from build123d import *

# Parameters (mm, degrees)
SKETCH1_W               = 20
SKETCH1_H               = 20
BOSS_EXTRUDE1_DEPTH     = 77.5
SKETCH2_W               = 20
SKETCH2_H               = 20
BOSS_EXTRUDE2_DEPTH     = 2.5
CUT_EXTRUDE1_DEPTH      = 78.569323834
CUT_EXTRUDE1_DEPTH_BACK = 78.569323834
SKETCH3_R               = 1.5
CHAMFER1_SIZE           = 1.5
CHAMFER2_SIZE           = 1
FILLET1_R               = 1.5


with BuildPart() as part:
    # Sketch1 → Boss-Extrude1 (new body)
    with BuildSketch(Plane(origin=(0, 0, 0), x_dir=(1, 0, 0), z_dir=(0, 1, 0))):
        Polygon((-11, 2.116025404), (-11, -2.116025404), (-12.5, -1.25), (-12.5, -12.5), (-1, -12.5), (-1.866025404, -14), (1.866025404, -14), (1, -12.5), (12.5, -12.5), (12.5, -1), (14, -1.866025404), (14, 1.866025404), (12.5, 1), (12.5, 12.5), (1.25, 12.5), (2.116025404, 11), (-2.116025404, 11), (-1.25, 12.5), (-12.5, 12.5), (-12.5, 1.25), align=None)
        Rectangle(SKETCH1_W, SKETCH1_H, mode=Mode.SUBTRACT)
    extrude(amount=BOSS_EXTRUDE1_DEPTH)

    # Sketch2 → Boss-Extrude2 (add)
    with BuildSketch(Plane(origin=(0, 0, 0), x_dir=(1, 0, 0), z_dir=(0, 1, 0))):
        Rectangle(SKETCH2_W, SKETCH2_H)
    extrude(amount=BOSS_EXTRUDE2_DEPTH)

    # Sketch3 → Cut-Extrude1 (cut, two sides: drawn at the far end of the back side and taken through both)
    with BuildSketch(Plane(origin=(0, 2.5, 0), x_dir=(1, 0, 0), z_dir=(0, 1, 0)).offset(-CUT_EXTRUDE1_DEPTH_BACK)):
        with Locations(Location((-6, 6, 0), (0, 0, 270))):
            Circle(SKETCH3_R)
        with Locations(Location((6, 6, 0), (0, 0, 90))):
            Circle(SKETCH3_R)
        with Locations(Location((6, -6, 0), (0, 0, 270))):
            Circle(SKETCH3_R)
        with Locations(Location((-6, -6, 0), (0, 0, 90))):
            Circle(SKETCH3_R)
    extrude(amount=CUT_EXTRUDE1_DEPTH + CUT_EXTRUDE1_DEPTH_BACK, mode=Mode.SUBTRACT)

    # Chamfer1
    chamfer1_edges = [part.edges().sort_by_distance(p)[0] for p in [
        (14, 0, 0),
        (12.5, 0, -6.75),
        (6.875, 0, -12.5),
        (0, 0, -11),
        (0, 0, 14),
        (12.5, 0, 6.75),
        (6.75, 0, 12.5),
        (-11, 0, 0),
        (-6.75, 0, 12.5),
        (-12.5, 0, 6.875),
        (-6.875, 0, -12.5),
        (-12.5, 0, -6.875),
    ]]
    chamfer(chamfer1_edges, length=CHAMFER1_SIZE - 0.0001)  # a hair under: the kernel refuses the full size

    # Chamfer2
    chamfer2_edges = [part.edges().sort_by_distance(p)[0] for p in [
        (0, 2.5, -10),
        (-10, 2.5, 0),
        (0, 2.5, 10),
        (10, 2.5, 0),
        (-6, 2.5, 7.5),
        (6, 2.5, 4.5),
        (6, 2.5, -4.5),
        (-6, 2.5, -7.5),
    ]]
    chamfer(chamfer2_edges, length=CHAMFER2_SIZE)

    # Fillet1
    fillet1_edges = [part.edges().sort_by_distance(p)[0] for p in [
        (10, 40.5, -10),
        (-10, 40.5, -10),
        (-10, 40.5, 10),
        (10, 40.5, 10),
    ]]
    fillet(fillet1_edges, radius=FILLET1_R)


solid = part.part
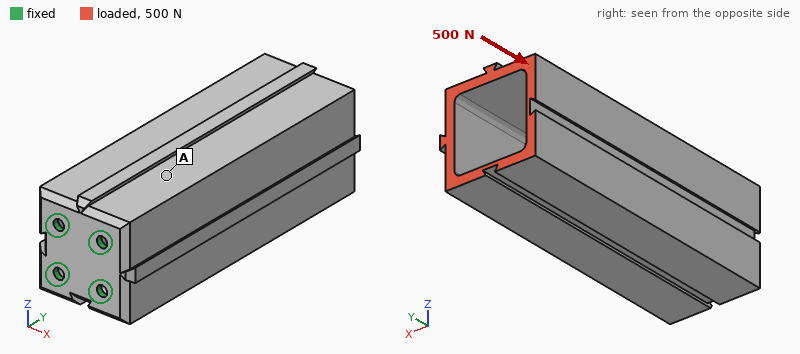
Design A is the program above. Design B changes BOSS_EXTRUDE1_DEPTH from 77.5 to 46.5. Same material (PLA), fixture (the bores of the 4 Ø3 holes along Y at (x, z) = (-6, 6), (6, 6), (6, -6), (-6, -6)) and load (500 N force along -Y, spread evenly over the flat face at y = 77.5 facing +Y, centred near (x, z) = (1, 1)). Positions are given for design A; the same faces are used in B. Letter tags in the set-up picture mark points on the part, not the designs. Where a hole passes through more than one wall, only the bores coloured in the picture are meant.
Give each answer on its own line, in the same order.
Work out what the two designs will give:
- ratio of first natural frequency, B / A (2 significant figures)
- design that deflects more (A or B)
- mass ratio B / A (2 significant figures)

2.1
A
0.62
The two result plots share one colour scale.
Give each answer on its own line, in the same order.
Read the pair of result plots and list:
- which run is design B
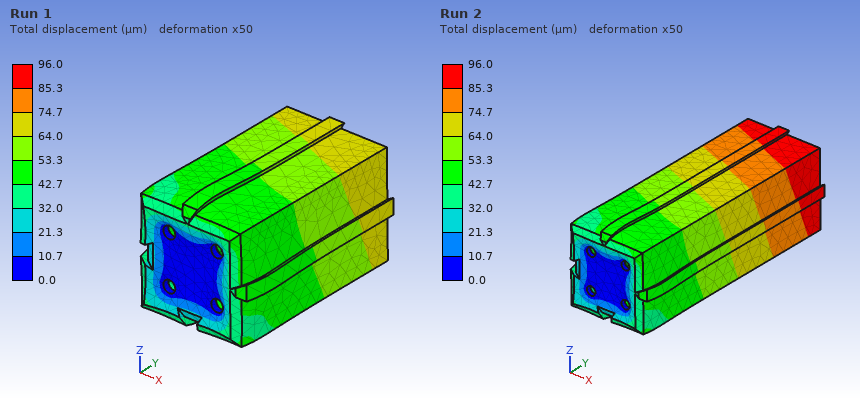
Run 1
